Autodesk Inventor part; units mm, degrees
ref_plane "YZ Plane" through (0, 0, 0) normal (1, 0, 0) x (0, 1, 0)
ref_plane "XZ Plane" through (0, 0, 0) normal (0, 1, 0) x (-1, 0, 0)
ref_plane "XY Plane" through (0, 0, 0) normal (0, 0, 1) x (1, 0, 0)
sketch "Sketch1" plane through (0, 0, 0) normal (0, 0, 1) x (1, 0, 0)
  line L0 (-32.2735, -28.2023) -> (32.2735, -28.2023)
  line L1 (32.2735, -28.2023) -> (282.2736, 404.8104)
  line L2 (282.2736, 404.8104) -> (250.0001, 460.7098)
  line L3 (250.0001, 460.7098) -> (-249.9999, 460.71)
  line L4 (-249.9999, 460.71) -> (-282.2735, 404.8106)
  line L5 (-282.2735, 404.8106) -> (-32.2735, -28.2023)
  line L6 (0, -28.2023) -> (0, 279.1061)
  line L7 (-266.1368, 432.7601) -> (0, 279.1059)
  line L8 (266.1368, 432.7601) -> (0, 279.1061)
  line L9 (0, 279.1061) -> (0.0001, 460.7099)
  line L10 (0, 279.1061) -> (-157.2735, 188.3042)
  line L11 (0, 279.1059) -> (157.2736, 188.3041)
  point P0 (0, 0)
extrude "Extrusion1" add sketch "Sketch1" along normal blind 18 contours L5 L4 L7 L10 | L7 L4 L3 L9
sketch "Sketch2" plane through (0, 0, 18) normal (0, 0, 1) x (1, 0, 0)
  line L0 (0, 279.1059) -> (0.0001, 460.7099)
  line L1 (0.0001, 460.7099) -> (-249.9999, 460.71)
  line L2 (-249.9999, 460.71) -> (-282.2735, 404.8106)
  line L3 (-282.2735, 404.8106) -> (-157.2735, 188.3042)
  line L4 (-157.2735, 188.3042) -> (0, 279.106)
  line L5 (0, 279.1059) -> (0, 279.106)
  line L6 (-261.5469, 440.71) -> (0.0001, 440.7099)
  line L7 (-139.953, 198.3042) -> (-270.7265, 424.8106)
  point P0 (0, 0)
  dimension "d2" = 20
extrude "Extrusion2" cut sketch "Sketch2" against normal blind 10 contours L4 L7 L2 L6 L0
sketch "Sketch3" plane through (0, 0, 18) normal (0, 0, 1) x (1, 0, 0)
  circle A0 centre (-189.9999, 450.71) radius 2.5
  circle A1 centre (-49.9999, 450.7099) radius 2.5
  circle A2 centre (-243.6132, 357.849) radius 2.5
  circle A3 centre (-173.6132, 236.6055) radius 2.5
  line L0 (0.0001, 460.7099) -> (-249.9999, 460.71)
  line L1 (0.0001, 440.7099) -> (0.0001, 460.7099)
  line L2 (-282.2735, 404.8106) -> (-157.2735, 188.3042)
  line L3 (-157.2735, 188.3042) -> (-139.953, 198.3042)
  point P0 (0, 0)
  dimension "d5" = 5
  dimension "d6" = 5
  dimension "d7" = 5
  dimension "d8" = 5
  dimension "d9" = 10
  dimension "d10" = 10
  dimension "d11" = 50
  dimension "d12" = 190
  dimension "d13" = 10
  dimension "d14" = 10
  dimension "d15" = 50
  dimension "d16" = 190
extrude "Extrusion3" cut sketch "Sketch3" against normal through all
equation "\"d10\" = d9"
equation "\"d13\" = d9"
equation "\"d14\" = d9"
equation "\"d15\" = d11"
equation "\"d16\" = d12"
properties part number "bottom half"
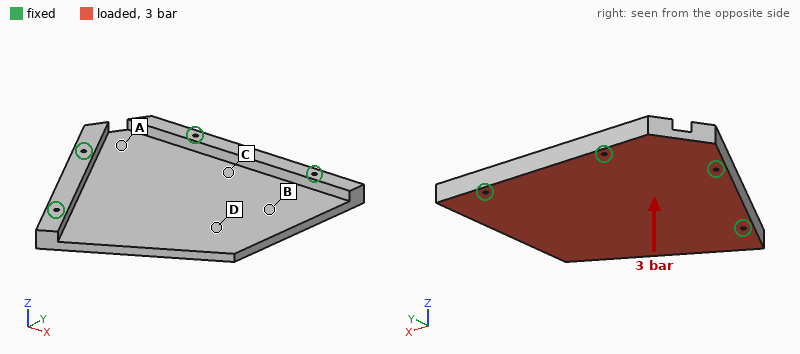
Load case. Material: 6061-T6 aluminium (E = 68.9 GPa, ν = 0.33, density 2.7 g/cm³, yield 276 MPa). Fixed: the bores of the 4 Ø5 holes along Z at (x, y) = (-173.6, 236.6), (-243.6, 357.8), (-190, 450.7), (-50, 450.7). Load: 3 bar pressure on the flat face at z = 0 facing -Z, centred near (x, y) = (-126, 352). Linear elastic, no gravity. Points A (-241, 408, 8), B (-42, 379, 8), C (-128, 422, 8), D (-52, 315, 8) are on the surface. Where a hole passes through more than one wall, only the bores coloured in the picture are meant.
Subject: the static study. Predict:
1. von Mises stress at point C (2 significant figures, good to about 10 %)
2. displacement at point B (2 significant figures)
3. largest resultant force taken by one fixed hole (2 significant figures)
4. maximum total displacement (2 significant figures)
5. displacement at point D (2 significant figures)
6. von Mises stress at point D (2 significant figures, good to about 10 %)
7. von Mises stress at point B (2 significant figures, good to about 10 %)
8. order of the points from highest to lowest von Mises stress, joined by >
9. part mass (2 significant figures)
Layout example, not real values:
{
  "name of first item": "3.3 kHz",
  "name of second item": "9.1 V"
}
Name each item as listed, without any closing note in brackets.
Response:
{
  "von Mises stress at point C": "39 MPa",
  "displacement at point B": "1.1 mm",
  "largest resultant force taken by one fixed hole": "7.2 kN",
  "maximum total displacement": "3.5 mm",
  "displacement at point D": "2.1 mm",
  "von Mises stress at point D": "72 MPa",
  "von Mises stress at point B": "51 MPa",
  "order of the points from highest to lowest von Mises stress, joined by >": "D > B > C > A",
  "part mass": "1.5 kg"
}
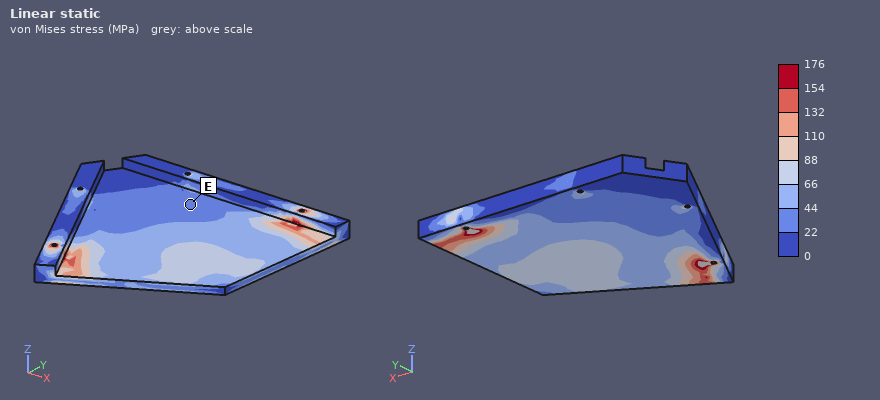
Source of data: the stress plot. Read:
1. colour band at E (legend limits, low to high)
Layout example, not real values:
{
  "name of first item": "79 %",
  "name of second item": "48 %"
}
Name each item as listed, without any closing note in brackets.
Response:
{
  "colour band at E": "22 to 44 MPa"
}
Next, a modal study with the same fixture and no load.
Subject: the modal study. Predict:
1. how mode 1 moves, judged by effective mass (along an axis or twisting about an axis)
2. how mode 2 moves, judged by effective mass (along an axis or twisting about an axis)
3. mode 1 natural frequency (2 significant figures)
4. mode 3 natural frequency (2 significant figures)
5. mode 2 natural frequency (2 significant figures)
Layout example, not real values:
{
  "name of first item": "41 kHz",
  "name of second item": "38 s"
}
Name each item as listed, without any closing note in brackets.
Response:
{
  "how mode 1 moves, judged by effective mass": "along Z",
  "how mode 2 moves, judged by effective mass": "along Z",
  "mode 1 natural frequency": "450 Hz",
  "mode 3 natural frequency": "1300 Hz",
  "mode 2 natural frequency": "1300 Hz"
}
